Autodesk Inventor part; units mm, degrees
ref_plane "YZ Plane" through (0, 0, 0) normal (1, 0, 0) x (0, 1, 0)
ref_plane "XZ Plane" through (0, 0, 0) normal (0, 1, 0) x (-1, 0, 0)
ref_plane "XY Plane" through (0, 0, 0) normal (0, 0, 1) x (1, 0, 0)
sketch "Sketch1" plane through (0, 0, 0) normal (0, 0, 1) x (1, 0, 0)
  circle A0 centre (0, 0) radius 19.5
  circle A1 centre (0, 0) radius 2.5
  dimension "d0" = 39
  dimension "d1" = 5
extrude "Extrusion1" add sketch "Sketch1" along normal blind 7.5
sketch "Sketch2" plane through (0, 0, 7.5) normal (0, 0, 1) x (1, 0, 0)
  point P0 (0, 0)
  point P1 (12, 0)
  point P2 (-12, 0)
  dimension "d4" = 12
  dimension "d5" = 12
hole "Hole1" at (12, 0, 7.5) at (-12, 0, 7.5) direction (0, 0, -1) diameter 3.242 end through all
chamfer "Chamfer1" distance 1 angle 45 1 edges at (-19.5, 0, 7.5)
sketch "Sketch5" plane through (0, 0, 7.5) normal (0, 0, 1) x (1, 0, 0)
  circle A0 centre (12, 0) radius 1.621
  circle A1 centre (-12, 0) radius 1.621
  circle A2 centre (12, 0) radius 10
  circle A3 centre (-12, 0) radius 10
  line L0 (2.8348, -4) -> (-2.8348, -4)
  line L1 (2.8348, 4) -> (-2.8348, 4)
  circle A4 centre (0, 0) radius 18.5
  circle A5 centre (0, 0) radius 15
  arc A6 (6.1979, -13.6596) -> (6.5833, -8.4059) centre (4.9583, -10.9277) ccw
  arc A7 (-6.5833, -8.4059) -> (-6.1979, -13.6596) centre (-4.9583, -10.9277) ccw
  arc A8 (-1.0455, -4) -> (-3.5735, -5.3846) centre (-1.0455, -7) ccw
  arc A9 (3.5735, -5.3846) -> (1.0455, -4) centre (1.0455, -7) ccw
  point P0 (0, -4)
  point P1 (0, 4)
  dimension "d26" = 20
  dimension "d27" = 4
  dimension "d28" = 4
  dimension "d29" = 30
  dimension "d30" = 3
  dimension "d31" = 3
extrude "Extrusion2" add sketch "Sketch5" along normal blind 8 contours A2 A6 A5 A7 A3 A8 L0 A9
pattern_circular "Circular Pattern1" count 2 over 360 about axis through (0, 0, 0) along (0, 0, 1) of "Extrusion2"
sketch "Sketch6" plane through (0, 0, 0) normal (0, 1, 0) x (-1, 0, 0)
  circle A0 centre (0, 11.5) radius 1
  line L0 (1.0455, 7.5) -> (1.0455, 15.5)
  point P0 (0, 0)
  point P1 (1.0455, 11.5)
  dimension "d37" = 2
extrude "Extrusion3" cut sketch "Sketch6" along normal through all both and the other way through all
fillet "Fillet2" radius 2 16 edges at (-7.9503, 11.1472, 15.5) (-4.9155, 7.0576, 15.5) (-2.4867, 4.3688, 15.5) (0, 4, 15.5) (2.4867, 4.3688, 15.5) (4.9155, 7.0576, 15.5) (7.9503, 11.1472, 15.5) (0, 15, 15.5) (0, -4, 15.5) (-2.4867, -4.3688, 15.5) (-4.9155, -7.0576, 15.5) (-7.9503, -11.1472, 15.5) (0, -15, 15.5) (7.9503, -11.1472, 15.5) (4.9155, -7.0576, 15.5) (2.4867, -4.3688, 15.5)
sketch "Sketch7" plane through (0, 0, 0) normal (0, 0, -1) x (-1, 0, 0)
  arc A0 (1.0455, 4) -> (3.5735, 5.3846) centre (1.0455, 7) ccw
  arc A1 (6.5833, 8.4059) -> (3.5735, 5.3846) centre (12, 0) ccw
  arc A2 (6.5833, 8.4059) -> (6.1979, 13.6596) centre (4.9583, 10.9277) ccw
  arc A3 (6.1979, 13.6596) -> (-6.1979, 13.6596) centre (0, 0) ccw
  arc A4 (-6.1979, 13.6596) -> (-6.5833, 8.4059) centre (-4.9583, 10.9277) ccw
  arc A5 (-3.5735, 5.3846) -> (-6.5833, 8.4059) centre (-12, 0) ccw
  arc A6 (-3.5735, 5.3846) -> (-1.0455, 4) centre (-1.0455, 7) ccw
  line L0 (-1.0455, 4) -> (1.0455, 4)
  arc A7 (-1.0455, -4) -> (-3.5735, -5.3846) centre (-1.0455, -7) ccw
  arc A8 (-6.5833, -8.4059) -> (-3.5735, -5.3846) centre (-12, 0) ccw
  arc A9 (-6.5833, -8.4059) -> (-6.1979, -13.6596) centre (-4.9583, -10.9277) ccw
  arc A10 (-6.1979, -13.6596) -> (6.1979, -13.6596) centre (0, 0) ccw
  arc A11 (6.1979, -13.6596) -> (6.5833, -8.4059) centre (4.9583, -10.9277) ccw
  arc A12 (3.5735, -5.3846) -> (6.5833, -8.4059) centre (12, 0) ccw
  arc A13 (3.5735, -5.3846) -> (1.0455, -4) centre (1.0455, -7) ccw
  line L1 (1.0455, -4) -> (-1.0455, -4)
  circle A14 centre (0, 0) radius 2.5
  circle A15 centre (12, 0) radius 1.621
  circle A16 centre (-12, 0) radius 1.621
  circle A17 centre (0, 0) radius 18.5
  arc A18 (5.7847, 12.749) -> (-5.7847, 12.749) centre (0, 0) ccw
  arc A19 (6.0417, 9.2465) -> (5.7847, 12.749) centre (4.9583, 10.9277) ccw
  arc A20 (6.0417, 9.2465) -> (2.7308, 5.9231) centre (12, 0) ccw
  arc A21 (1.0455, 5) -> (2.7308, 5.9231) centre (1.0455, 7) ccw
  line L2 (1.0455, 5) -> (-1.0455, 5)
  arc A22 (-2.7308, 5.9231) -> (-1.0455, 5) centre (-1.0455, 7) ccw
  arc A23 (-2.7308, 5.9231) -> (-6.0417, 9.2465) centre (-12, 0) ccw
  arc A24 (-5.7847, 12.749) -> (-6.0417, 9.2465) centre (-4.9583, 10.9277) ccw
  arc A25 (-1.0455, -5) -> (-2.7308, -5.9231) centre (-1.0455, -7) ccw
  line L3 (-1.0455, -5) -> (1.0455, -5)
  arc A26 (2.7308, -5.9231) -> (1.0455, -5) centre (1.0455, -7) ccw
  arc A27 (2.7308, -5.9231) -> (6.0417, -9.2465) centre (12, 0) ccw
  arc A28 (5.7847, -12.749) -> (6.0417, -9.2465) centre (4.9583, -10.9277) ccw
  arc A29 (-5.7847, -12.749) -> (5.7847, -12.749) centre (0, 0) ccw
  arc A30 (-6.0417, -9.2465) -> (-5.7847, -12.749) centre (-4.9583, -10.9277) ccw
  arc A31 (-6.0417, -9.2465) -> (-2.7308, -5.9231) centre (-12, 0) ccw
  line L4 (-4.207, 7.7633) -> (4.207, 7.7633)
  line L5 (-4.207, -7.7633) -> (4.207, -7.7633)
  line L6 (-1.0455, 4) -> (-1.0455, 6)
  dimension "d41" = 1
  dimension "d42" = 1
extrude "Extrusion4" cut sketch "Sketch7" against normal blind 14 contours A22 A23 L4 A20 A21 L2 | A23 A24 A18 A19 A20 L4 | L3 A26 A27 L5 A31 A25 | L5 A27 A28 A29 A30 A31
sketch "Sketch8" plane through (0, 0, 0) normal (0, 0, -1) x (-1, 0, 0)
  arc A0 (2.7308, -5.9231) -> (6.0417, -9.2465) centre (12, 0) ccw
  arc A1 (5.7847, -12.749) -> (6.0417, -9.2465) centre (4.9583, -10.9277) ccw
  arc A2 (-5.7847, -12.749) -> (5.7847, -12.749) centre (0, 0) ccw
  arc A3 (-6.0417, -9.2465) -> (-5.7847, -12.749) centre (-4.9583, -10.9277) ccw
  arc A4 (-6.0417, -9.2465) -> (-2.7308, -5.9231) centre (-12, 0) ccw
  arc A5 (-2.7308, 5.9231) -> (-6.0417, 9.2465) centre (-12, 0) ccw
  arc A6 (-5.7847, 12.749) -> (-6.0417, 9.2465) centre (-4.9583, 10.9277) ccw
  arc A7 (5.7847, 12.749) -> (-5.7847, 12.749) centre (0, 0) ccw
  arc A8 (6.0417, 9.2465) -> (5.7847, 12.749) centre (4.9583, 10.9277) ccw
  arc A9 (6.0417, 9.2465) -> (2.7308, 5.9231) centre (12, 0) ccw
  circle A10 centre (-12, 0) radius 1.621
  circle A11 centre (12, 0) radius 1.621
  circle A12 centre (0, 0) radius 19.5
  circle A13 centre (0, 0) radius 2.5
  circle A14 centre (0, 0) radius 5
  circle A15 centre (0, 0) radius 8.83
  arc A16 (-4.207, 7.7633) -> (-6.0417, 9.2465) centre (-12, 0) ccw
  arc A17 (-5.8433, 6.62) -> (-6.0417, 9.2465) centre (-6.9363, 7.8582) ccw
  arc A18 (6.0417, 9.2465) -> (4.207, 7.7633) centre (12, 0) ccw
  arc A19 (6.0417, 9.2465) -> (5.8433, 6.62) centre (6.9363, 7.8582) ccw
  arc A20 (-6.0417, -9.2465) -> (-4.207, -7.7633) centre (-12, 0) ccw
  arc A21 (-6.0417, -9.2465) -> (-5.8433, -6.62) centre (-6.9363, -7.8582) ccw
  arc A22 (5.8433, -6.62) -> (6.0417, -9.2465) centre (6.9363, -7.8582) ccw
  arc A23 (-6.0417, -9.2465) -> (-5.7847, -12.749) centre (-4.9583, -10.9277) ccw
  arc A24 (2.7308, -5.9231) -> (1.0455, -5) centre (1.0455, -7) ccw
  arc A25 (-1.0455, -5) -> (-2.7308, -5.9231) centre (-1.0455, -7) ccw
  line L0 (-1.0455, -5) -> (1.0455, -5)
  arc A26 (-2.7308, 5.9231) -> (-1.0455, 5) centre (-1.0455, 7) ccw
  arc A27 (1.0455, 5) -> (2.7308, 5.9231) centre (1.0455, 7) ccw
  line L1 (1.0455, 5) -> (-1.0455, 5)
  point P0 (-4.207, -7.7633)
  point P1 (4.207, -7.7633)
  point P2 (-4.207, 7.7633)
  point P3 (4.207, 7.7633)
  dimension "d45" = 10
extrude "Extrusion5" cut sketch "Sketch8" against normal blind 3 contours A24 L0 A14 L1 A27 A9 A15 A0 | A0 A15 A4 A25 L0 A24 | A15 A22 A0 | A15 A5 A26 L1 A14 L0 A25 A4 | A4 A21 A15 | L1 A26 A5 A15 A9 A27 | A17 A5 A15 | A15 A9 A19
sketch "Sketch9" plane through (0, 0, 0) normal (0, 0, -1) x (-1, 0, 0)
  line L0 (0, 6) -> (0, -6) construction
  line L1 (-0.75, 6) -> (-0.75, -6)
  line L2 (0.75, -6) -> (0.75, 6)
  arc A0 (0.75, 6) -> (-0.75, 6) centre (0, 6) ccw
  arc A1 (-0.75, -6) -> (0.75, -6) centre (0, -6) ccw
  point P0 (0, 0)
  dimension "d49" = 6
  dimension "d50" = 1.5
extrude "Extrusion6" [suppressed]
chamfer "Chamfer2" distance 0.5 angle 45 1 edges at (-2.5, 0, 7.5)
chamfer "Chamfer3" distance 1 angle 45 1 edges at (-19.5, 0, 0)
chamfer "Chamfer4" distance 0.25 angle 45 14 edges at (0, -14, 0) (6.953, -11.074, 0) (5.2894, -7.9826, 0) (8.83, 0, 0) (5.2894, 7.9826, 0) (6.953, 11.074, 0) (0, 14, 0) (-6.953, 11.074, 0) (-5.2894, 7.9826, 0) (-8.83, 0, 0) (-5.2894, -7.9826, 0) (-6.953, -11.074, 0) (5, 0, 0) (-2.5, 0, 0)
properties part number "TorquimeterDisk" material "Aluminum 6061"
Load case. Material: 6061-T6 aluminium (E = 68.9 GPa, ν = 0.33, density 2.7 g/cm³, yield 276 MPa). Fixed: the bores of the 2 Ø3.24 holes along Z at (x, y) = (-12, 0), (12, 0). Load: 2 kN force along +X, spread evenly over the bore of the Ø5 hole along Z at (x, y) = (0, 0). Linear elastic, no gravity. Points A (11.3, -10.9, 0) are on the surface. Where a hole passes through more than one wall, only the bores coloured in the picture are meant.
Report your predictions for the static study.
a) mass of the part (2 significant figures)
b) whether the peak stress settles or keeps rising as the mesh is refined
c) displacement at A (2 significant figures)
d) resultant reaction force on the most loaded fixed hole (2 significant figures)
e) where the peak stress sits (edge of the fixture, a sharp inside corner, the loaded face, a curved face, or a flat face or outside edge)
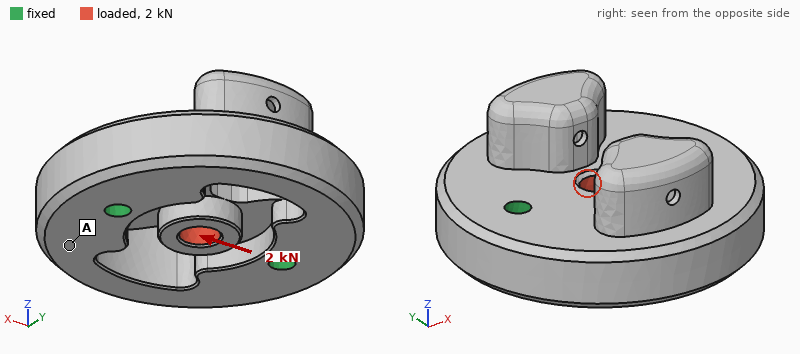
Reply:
21 g
keeps rising
1.0 µm
1.0 kN
edge of the fixture
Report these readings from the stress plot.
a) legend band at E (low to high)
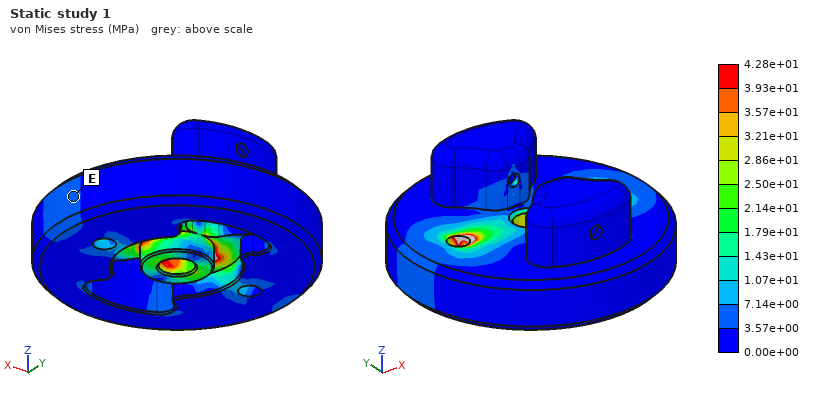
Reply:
3.57e+00 to 7.14e+00 MPa
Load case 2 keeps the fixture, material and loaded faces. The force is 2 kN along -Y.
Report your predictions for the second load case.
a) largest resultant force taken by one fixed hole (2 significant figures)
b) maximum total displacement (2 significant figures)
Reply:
1.0 kN
12 µm
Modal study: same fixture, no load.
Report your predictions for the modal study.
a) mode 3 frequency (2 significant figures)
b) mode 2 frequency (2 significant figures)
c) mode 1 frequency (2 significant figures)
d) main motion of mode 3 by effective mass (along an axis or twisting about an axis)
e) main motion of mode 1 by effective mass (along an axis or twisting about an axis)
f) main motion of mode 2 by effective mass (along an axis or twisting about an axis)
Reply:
22 kHz
15 kHz
13 kHz
twisting about Z
twisting about X
along Z
